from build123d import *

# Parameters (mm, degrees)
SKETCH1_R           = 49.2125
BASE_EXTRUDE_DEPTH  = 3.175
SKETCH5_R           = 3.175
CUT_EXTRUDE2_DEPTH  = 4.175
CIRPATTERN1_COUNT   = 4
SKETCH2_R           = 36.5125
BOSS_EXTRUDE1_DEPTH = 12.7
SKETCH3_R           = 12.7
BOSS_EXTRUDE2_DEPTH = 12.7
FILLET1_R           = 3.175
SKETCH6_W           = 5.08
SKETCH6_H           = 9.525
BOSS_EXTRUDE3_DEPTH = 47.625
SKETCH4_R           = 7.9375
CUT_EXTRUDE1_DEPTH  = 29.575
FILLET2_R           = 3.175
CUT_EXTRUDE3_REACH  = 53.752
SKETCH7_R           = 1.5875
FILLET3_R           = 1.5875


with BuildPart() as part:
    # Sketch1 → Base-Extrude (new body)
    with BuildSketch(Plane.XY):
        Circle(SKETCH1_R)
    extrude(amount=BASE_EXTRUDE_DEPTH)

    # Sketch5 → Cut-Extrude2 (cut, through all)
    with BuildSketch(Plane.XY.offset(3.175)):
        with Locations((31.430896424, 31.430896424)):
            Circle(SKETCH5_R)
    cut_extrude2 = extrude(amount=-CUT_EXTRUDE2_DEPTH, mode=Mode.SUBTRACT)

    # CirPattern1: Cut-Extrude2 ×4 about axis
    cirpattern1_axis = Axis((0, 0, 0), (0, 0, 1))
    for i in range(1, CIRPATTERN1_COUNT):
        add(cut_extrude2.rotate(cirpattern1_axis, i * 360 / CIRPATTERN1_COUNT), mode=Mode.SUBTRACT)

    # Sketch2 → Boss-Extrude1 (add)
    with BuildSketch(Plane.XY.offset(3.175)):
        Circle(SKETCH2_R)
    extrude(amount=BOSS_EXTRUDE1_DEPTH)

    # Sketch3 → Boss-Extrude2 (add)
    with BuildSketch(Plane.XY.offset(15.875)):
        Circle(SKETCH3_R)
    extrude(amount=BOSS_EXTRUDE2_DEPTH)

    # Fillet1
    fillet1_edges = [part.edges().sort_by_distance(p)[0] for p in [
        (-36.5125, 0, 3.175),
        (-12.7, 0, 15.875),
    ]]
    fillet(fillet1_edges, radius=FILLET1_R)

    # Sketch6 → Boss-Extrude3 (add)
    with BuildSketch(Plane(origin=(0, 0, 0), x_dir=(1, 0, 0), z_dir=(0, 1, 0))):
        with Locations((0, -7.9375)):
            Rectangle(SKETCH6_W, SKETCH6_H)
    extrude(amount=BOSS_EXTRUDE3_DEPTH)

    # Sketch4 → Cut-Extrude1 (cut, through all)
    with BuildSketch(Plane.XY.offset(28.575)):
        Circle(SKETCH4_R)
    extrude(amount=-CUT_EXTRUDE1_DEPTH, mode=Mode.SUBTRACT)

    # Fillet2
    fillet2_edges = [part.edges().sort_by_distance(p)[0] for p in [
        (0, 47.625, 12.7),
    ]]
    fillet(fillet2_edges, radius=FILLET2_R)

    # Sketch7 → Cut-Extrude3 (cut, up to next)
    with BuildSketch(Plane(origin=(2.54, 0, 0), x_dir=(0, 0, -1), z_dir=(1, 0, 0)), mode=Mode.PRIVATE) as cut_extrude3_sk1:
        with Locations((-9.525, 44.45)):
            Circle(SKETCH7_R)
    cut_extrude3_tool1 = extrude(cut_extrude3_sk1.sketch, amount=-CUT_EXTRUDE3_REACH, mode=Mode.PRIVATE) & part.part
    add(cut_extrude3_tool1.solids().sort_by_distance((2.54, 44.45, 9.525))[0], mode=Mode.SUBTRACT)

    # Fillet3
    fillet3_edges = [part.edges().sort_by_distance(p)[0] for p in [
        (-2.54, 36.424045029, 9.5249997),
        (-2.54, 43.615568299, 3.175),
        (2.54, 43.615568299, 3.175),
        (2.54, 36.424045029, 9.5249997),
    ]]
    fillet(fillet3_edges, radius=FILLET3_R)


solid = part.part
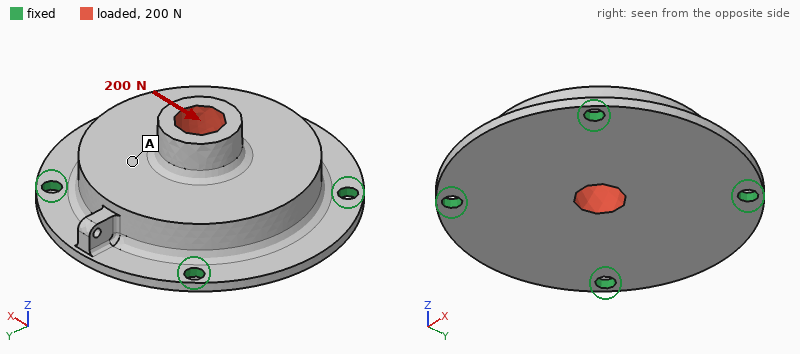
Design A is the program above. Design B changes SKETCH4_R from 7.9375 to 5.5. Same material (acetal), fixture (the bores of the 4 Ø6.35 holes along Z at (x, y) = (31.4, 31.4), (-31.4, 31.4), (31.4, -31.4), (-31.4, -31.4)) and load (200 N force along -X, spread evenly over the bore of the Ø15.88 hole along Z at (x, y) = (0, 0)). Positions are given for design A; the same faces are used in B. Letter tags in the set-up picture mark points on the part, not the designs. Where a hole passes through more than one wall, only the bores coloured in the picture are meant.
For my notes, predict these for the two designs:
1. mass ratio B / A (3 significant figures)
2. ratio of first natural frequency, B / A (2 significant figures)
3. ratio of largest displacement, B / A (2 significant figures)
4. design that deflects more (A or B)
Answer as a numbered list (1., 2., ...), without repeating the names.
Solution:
1. 1.04
2. 0.98
3. 0.91
4. A
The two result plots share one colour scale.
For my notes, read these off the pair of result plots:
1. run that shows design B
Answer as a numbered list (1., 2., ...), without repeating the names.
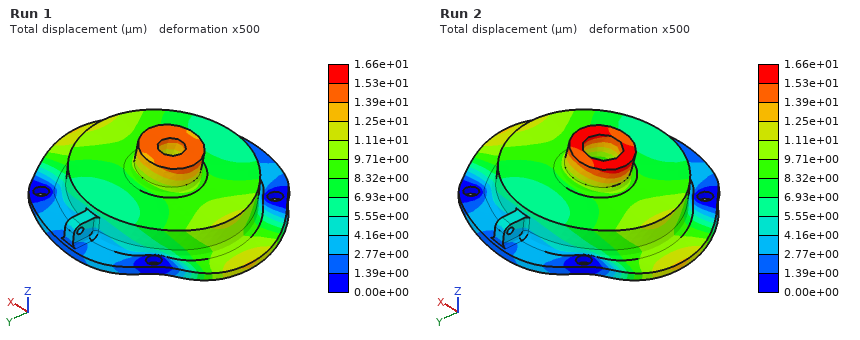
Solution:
1. Run 1
